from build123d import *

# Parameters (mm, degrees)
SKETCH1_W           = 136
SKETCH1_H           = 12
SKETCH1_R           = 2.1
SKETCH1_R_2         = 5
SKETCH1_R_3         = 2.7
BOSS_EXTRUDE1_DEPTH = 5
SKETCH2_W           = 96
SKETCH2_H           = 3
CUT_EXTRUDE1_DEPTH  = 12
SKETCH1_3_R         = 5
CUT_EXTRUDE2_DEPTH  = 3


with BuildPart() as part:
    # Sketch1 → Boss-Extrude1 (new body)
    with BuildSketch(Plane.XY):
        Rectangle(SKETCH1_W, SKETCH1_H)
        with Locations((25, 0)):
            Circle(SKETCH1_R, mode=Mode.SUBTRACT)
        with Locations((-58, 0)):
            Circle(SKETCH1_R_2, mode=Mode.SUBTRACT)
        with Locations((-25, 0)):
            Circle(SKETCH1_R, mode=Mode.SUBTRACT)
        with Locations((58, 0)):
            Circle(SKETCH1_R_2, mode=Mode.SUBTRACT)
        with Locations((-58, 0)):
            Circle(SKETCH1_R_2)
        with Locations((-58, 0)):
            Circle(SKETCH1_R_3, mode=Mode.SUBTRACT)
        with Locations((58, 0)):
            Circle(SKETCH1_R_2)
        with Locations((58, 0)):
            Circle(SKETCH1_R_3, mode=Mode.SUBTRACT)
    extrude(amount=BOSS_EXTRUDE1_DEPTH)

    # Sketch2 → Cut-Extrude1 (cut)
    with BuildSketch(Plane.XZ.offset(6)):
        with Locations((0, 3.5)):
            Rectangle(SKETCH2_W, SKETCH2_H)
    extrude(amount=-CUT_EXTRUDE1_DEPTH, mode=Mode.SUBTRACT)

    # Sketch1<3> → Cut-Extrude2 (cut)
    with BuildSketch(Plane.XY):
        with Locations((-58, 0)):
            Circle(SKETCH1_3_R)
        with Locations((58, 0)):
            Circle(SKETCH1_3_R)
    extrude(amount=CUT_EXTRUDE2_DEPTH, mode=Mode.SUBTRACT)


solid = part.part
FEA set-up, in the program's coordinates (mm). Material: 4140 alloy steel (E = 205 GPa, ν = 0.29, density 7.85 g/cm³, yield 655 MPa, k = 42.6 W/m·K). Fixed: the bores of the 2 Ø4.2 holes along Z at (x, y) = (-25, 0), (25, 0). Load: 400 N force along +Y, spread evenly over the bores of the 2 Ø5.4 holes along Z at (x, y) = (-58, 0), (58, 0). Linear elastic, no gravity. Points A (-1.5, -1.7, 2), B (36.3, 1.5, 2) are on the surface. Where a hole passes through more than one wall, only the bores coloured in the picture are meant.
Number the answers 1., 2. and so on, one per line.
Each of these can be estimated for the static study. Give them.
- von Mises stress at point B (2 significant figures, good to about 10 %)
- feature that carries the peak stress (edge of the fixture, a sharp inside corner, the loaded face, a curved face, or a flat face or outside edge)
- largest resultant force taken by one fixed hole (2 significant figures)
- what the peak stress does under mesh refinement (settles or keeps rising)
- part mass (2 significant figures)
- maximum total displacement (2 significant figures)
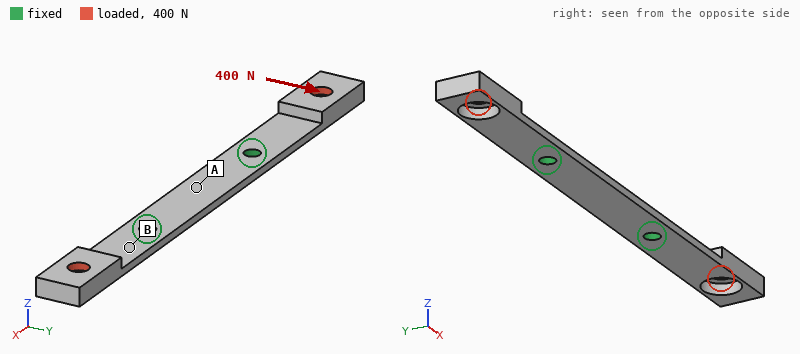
1. 93 MPa
2. edge of the fixture
3. 200 N
4. keeps rising
5. 32 g
6. 0.11 mm
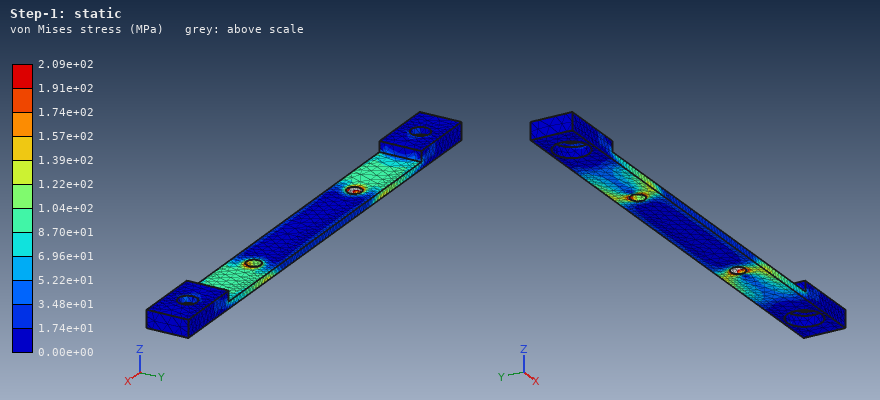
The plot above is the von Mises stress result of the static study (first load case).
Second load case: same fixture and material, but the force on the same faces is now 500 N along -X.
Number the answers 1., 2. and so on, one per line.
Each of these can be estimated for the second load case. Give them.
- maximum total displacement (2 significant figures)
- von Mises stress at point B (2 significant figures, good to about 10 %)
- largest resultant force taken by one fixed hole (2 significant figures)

1. 0.31 mm
2. 100 MPa
3. 250 N
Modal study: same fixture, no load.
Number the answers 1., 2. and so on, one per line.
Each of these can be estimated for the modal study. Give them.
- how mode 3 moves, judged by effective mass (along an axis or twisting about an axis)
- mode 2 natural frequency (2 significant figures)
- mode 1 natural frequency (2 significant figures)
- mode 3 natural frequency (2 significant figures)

1. along Y
2. 700 Hz
3. 700 Hz
4. 3100 Hz
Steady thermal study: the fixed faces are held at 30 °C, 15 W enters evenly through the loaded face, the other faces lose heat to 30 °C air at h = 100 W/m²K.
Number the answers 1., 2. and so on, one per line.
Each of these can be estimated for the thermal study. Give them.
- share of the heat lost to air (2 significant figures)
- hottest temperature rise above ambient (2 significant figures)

1. 79 %
2. 73 K
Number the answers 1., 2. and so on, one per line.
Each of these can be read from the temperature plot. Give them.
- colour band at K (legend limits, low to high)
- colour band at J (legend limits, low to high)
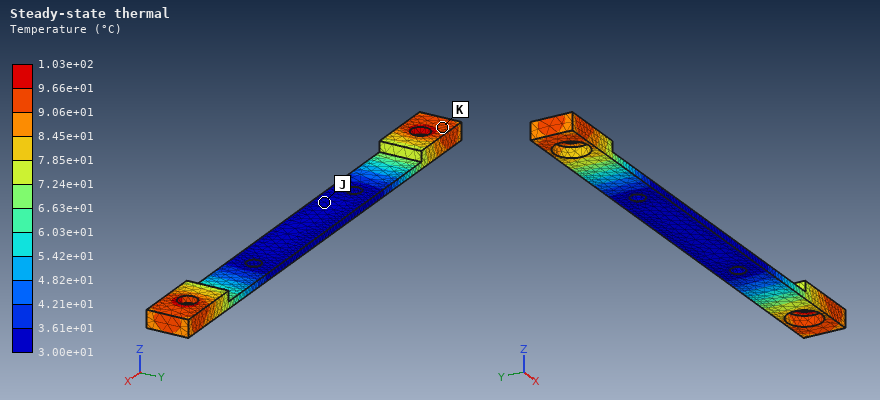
1. 9.06e+01 to 9.66e+01 °C
2. 3.00e+01 to 3.61e+01 °C
